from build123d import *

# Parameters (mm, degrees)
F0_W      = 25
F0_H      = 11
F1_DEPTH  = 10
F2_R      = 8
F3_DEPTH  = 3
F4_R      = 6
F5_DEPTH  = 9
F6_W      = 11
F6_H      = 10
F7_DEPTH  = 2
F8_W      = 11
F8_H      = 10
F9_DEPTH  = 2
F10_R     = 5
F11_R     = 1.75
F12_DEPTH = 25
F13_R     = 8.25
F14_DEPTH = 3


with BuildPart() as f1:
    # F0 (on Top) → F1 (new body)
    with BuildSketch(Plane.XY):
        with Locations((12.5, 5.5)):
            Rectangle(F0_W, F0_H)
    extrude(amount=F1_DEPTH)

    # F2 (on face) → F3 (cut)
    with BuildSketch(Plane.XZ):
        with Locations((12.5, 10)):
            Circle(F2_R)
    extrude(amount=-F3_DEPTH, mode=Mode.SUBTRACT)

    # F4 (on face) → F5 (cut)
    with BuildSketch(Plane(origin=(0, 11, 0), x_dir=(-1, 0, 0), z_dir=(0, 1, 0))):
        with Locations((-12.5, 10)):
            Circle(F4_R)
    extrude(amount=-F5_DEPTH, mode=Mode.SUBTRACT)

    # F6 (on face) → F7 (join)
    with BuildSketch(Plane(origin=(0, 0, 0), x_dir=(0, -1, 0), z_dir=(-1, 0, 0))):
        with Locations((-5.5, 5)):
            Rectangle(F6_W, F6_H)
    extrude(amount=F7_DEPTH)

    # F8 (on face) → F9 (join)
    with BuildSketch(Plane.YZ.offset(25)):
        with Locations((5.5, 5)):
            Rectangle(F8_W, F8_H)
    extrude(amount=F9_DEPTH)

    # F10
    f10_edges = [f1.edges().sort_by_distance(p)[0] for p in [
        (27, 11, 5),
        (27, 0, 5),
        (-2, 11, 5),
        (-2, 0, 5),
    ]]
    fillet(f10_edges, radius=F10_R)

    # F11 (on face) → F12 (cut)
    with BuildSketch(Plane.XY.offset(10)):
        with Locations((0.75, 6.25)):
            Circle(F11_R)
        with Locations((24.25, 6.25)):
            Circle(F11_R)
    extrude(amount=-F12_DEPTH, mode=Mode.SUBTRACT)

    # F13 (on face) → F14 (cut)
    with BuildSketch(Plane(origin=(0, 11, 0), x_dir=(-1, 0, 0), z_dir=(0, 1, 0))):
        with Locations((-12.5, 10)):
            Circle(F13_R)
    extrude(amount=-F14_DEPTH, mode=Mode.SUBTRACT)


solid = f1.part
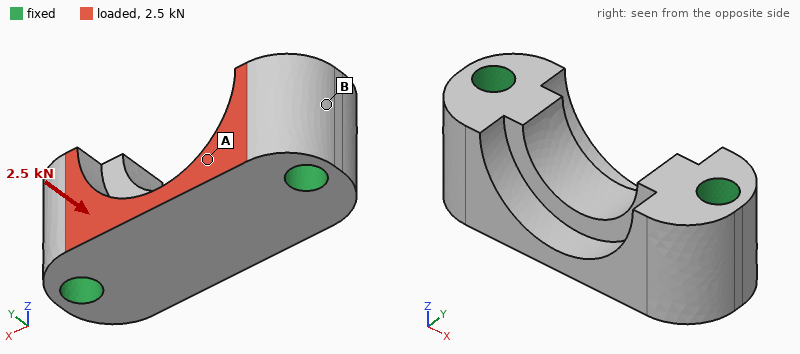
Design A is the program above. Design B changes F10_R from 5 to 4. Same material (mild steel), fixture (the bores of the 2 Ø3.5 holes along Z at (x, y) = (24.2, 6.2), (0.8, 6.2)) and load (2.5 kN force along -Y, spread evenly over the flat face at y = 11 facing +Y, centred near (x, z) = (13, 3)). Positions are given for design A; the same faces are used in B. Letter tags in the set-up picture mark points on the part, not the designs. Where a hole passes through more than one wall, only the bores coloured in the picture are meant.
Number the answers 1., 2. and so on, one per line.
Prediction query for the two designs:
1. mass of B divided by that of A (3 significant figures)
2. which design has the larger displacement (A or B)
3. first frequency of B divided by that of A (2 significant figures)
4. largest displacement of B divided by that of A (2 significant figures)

1. 1.04
2. A
3. 1.0
4. 0.82
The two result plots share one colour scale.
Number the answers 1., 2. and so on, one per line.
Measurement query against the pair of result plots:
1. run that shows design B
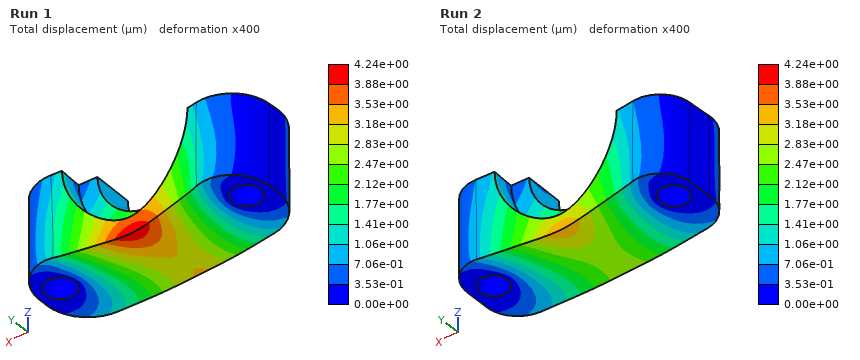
1. Run 2
